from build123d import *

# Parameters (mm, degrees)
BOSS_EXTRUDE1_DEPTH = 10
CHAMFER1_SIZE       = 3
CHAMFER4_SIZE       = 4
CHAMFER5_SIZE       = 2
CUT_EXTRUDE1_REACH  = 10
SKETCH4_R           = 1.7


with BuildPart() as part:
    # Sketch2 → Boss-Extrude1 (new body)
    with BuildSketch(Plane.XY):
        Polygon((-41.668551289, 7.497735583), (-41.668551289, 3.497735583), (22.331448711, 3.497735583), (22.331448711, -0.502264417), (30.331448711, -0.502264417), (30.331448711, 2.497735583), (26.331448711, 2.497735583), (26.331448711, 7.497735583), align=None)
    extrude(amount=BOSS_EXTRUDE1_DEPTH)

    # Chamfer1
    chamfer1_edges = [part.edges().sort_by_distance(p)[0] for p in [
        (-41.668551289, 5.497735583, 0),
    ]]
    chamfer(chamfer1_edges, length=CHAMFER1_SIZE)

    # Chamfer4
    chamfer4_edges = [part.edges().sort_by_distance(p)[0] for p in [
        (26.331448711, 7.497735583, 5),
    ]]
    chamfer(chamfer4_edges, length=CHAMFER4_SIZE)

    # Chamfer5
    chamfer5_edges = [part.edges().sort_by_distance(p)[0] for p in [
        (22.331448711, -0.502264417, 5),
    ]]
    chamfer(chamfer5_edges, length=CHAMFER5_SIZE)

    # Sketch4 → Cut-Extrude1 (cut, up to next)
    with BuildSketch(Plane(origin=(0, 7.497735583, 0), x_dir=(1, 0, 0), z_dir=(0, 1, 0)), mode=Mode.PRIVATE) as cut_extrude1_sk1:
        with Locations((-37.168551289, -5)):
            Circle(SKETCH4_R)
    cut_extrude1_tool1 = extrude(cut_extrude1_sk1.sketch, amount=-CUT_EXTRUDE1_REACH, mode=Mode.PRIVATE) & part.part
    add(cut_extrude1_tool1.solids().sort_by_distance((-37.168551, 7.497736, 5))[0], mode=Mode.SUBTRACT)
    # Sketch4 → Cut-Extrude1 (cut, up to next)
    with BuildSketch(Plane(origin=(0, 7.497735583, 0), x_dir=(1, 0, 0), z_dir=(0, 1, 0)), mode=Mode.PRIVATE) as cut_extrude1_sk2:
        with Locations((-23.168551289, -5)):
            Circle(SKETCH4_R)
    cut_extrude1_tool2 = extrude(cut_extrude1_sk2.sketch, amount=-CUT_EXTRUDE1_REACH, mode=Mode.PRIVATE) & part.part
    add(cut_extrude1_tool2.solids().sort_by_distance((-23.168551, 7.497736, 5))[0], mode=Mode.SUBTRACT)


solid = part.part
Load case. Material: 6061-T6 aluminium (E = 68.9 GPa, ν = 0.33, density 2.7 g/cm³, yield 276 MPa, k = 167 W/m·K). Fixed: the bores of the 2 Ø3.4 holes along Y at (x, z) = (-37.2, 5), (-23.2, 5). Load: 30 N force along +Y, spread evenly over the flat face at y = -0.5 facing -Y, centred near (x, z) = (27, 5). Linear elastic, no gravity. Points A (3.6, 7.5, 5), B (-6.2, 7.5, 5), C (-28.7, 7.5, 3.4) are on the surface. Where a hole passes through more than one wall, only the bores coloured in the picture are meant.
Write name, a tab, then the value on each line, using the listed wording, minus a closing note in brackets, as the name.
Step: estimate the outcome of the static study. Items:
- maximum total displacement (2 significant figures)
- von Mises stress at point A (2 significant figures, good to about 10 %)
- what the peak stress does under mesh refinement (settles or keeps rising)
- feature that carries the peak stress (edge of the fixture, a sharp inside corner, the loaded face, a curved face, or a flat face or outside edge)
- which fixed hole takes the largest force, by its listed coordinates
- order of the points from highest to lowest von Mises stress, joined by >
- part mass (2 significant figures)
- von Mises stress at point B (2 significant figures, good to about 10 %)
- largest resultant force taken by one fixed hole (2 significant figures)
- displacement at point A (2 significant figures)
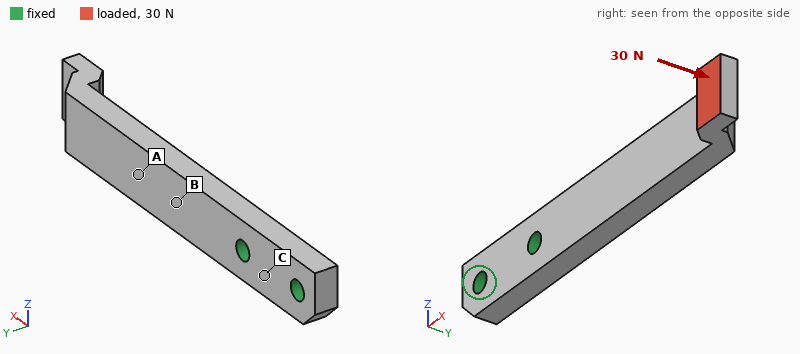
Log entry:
maximum total displacement	0.37 mm
von Mises stress at point A	27 MPa
what the peak stress does under mesh refinement	keeps rising
feature that carries the peak stress	edge of the fixture
which fixed hole takes the largest force, by its listed coordinates	(-23.2, 5)
order of the points from highest to lowest von Mises stress, joined by >	B > A > C
part mass	7.6 g
von Mises stress at point B	38 MPa
largest resultant force taken by one fixed hole	42 N
displacement at point A	0.12 mm
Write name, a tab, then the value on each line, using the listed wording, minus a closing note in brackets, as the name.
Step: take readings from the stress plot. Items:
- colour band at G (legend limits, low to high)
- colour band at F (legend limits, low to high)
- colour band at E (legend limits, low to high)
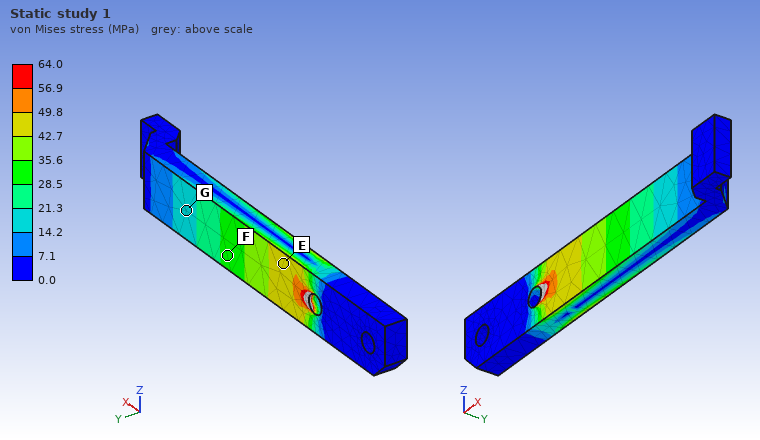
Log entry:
colour band at G	14.2 to 21.3 MPa
colour band at F	28.5 to 35.6 MPa
colour band at E	42.7 to 49.8 MPa
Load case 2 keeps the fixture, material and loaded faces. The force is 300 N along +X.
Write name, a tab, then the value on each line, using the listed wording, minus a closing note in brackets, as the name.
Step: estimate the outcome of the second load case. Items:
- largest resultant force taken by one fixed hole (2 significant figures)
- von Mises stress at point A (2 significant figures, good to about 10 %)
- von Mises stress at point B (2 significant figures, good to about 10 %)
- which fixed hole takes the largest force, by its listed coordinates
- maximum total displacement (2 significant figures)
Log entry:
largest resultant force taken by one fixed hole	280 N
von Mises stress at point A	60 MPa
von Mises stress at point B	60 MPa
which fixed hole takes the largest force, by its listed coordinates	(-23.2, 5)
maximum total displacement	0.70 mm
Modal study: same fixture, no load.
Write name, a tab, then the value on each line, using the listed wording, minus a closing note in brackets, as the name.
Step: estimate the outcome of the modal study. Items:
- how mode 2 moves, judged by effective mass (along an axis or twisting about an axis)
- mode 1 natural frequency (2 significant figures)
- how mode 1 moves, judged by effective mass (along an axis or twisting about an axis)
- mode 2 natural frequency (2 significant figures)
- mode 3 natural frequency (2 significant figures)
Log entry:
how mode 2 moves, judged by effective mass	along Z
mode 1 natural frequency	1200 Hz
how mode 1 moves, judged by effective mass	along Y
mode 2 natural frequency	2500 Hz
mode 3 natural frequency	7000 Hz
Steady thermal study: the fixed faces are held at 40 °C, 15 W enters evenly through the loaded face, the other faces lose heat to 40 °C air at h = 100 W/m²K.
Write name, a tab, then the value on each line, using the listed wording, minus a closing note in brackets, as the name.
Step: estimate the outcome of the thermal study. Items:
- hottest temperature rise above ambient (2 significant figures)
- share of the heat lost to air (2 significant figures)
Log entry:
hottest temperature rise above ambient	87 K
share of the heat lost to air	40 %
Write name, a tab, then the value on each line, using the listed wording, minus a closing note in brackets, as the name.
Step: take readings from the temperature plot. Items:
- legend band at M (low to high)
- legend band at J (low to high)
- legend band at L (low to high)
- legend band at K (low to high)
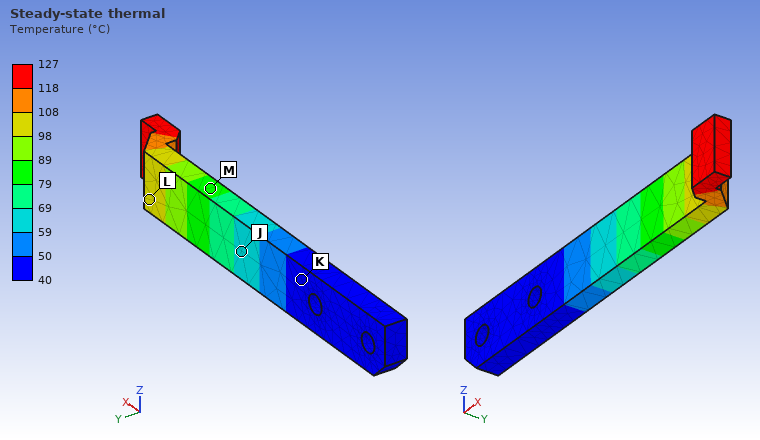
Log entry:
legend band at M	79 to 89 °C
legend band at J	59 to 69 °C
legend band at L	98 to 108 °C
legend band at K	40 to 50 °C
